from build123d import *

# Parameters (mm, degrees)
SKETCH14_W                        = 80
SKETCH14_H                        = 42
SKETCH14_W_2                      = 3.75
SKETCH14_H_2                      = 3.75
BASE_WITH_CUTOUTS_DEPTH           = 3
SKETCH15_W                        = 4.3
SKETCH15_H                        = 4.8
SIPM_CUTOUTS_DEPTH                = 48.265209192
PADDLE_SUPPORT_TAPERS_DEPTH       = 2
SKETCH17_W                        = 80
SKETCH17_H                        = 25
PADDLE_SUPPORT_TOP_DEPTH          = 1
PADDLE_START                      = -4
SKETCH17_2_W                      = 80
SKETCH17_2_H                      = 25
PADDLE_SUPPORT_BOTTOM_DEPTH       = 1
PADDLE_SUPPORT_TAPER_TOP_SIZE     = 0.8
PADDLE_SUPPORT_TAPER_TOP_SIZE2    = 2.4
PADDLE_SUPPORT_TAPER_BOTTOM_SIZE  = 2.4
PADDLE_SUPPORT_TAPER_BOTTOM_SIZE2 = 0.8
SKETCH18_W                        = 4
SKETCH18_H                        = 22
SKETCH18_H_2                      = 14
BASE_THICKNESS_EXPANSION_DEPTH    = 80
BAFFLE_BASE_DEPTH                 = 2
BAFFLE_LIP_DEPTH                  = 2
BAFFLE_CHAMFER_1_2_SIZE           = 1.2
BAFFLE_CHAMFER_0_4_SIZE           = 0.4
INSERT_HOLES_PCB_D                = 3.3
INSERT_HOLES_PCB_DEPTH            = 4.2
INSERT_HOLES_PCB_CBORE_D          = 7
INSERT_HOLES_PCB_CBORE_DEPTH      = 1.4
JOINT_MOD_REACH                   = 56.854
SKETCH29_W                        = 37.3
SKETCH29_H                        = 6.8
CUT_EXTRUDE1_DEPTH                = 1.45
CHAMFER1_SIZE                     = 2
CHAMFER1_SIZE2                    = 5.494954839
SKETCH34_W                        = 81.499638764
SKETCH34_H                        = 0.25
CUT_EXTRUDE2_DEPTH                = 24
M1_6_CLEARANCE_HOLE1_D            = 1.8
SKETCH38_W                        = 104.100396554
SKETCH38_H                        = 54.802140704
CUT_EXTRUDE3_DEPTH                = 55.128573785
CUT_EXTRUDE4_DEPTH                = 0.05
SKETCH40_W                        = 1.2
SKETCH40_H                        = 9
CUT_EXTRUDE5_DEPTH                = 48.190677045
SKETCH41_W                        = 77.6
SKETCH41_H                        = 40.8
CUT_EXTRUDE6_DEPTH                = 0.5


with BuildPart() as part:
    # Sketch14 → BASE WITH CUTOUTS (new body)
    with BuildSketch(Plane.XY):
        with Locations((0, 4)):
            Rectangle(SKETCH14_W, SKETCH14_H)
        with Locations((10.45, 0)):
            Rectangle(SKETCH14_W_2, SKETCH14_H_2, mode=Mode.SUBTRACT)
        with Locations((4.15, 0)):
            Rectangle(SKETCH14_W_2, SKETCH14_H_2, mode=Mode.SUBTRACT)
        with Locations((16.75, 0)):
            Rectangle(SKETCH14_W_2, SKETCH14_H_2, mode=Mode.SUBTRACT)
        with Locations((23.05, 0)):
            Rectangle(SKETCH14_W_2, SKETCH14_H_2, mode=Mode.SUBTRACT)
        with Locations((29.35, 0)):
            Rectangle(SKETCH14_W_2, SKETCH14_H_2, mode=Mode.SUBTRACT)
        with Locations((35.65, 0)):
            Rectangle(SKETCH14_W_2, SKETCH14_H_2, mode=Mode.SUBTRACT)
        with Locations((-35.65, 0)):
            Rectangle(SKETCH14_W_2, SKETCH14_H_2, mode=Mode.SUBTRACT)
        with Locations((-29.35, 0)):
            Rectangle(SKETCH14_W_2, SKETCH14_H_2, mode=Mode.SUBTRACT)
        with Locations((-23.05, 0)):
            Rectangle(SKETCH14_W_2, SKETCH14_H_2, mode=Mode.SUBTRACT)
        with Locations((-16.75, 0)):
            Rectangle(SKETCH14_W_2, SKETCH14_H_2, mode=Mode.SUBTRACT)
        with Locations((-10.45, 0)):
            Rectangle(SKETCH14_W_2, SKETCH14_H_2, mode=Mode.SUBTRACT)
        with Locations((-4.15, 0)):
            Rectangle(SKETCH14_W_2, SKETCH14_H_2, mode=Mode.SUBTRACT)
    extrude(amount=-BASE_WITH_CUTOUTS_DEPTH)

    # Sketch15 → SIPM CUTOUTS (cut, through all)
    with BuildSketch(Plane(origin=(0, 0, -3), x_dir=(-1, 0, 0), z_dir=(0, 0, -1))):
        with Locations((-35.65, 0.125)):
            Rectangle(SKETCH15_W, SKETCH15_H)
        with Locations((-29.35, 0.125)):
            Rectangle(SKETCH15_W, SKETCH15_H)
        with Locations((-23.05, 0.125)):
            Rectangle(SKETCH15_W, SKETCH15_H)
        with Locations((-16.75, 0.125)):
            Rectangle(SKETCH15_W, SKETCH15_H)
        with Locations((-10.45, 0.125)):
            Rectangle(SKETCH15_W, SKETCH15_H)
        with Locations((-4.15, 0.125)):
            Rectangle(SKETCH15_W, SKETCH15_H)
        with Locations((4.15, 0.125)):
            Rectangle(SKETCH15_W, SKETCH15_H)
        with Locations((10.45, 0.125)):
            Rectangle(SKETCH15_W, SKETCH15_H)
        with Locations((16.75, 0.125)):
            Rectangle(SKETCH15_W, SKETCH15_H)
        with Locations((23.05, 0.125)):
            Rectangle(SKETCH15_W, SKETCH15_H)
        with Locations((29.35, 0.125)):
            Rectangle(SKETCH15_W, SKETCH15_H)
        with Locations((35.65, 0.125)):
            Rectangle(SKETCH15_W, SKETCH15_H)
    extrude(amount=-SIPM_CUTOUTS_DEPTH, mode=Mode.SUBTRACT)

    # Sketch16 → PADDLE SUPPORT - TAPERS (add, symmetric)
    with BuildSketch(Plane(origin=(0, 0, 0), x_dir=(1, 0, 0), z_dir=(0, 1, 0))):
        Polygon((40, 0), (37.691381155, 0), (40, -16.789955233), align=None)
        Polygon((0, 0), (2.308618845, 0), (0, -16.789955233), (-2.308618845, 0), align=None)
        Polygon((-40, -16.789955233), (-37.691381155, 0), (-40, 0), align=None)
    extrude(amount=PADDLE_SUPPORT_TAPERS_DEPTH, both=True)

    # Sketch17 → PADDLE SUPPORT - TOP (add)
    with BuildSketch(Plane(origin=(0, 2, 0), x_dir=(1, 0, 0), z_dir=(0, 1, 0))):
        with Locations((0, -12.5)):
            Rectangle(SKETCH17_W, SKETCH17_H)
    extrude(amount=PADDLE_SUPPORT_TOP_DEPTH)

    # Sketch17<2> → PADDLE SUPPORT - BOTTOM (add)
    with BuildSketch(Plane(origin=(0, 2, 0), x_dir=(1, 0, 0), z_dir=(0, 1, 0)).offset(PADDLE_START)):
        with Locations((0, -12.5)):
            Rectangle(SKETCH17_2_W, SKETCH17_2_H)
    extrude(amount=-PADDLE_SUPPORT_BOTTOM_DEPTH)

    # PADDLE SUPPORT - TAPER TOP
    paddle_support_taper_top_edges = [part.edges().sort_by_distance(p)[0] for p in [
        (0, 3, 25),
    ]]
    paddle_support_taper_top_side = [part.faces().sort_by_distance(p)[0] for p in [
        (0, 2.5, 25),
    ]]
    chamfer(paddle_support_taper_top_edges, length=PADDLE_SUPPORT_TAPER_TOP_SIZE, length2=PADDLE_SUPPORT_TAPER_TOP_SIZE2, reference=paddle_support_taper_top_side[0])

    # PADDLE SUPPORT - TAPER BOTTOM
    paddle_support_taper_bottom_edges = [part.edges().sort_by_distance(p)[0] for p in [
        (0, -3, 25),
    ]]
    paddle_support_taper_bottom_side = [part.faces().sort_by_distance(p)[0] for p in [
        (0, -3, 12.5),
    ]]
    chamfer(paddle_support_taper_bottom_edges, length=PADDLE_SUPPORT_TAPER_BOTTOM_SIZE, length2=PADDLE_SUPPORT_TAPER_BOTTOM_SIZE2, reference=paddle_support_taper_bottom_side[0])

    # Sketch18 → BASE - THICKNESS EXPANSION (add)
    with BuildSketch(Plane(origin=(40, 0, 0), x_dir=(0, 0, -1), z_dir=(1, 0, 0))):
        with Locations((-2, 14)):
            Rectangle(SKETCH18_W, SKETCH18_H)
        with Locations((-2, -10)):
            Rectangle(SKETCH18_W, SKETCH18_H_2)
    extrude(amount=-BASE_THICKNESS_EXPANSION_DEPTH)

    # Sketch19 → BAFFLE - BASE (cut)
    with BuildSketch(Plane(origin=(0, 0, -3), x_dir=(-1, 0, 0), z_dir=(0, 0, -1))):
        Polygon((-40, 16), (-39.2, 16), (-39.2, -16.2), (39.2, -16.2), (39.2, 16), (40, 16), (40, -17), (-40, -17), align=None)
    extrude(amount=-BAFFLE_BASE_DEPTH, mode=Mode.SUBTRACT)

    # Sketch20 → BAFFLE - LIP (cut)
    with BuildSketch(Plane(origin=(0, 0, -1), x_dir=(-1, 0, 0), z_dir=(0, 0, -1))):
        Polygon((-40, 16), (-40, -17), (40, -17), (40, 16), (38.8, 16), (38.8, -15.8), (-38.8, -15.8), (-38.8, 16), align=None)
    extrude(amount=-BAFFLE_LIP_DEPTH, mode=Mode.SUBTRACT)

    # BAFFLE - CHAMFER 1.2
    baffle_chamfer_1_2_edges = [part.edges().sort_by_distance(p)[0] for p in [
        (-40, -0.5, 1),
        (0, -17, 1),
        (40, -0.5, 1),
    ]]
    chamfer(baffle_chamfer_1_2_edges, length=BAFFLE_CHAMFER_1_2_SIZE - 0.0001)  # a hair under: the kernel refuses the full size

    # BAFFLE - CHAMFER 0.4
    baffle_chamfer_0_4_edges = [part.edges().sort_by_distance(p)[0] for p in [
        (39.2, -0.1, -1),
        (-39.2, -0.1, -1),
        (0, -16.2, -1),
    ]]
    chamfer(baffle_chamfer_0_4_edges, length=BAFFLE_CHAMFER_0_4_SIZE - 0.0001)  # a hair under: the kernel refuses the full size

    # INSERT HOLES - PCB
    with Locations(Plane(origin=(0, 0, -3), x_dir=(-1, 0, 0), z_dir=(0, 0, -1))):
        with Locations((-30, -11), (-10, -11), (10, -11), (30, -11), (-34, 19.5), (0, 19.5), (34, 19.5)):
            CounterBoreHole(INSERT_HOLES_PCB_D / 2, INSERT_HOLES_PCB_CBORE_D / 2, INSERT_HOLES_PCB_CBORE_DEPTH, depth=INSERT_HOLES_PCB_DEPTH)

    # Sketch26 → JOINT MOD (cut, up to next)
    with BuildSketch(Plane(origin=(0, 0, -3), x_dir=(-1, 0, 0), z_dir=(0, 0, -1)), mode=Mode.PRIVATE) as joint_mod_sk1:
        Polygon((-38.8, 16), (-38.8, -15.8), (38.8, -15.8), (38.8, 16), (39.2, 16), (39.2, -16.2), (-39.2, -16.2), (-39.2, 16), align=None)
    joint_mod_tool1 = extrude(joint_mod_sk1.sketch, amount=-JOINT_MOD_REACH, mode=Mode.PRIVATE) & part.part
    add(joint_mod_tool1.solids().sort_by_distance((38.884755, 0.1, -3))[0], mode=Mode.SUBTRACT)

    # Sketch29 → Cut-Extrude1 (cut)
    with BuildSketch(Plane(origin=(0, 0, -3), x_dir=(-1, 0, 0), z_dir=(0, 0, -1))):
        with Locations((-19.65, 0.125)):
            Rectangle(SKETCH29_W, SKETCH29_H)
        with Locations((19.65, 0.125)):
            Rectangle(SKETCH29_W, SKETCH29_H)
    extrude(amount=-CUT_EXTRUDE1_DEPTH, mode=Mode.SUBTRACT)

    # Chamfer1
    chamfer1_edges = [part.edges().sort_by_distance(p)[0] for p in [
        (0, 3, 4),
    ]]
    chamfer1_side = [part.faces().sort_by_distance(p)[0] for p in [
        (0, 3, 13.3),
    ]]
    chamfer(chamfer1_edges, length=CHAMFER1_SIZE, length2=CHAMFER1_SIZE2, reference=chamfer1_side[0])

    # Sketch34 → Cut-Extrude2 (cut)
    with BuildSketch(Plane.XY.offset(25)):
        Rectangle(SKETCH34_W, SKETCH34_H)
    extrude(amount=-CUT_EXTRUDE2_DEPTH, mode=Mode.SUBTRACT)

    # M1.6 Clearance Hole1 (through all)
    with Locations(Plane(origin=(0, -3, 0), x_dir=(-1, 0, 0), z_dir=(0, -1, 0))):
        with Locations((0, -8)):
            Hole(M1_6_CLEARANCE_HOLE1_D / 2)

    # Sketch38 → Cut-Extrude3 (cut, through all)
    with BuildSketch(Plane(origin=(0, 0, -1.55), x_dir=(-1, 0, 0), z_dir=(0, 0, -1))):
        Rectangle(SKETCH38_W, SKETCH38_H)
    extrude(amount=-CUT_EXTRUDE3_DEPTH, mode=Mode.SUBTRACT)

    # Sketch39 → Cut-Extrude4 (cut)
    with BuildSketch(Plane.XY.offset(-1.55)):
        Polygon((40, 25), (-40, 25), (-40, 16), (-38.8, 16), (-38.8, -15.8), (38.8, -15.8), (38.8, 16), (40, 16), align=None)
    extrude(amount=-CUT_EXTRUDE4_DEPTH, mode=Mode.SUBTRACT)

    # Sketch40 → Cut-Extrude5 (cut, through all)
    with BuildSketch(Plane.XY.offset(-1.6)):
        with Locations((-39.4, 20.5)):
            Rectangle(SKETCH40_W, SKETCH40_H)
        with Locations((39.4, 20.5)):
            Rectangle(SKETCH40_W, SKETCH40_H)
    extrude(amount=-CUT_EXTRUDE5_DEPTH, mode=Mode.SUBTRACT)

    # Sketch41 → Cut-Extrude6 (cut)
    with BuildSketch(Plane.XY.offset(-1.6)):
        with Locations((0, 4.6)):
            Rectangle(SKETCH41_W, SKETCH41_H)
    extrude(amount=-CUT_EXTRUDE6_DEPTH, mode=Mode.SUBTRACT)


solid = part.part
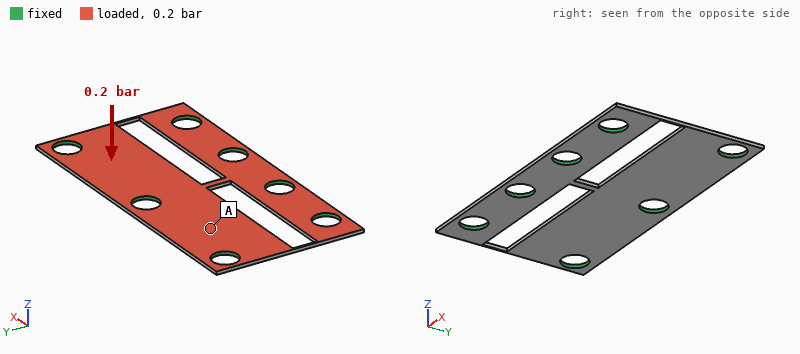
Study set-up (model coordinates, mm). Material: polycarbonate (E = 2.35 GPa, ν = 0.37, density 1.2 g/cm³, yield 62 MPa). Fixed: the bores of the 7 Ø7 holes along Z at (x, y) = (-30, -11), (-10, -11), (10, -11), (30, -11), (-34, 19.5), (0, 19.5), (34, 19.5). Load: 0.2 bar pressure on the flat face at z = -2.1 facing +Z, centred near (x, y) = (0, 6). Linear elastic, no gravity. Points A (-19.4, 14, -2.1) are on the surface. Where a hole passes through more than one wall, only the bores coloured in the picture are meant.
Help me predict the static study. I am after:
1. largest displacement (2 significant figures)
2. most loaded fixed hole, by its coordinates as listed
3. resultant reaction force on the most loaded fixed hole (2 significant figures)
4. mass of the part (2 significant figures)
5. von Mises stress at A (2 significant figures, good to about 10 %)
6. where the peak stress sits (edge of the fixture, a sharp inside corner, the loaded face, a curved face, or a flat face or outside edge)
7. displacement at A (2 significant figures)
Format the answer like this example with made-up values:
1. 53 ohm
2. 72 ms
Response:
1. 0.90 mm
2. (0, 19.5)
3. 13 N
4. 2.6 g
5. 5.6 MPa
6. a flat face or outside edge
7. 0.39 mm
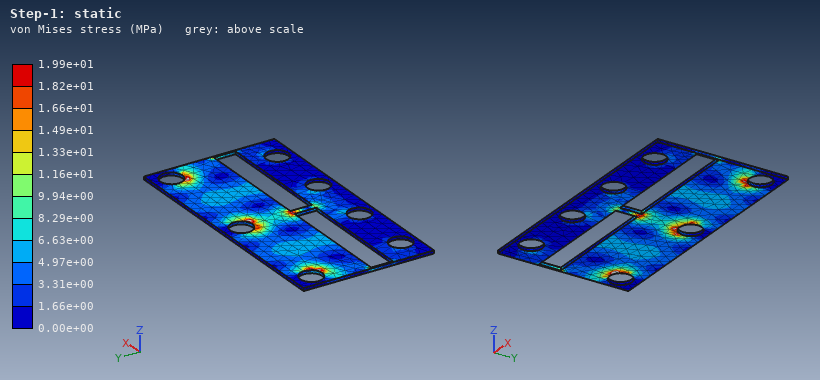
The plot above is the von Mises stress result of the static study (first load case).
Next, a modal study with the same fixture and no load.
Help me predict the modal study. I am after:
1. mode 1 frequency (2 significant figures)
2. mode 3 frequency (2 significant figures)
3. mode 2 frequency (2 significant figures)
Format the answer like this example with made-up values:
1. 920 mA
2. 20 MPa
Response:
1. 970 Hz
2. 1800 Hz
3. 980 Hz
